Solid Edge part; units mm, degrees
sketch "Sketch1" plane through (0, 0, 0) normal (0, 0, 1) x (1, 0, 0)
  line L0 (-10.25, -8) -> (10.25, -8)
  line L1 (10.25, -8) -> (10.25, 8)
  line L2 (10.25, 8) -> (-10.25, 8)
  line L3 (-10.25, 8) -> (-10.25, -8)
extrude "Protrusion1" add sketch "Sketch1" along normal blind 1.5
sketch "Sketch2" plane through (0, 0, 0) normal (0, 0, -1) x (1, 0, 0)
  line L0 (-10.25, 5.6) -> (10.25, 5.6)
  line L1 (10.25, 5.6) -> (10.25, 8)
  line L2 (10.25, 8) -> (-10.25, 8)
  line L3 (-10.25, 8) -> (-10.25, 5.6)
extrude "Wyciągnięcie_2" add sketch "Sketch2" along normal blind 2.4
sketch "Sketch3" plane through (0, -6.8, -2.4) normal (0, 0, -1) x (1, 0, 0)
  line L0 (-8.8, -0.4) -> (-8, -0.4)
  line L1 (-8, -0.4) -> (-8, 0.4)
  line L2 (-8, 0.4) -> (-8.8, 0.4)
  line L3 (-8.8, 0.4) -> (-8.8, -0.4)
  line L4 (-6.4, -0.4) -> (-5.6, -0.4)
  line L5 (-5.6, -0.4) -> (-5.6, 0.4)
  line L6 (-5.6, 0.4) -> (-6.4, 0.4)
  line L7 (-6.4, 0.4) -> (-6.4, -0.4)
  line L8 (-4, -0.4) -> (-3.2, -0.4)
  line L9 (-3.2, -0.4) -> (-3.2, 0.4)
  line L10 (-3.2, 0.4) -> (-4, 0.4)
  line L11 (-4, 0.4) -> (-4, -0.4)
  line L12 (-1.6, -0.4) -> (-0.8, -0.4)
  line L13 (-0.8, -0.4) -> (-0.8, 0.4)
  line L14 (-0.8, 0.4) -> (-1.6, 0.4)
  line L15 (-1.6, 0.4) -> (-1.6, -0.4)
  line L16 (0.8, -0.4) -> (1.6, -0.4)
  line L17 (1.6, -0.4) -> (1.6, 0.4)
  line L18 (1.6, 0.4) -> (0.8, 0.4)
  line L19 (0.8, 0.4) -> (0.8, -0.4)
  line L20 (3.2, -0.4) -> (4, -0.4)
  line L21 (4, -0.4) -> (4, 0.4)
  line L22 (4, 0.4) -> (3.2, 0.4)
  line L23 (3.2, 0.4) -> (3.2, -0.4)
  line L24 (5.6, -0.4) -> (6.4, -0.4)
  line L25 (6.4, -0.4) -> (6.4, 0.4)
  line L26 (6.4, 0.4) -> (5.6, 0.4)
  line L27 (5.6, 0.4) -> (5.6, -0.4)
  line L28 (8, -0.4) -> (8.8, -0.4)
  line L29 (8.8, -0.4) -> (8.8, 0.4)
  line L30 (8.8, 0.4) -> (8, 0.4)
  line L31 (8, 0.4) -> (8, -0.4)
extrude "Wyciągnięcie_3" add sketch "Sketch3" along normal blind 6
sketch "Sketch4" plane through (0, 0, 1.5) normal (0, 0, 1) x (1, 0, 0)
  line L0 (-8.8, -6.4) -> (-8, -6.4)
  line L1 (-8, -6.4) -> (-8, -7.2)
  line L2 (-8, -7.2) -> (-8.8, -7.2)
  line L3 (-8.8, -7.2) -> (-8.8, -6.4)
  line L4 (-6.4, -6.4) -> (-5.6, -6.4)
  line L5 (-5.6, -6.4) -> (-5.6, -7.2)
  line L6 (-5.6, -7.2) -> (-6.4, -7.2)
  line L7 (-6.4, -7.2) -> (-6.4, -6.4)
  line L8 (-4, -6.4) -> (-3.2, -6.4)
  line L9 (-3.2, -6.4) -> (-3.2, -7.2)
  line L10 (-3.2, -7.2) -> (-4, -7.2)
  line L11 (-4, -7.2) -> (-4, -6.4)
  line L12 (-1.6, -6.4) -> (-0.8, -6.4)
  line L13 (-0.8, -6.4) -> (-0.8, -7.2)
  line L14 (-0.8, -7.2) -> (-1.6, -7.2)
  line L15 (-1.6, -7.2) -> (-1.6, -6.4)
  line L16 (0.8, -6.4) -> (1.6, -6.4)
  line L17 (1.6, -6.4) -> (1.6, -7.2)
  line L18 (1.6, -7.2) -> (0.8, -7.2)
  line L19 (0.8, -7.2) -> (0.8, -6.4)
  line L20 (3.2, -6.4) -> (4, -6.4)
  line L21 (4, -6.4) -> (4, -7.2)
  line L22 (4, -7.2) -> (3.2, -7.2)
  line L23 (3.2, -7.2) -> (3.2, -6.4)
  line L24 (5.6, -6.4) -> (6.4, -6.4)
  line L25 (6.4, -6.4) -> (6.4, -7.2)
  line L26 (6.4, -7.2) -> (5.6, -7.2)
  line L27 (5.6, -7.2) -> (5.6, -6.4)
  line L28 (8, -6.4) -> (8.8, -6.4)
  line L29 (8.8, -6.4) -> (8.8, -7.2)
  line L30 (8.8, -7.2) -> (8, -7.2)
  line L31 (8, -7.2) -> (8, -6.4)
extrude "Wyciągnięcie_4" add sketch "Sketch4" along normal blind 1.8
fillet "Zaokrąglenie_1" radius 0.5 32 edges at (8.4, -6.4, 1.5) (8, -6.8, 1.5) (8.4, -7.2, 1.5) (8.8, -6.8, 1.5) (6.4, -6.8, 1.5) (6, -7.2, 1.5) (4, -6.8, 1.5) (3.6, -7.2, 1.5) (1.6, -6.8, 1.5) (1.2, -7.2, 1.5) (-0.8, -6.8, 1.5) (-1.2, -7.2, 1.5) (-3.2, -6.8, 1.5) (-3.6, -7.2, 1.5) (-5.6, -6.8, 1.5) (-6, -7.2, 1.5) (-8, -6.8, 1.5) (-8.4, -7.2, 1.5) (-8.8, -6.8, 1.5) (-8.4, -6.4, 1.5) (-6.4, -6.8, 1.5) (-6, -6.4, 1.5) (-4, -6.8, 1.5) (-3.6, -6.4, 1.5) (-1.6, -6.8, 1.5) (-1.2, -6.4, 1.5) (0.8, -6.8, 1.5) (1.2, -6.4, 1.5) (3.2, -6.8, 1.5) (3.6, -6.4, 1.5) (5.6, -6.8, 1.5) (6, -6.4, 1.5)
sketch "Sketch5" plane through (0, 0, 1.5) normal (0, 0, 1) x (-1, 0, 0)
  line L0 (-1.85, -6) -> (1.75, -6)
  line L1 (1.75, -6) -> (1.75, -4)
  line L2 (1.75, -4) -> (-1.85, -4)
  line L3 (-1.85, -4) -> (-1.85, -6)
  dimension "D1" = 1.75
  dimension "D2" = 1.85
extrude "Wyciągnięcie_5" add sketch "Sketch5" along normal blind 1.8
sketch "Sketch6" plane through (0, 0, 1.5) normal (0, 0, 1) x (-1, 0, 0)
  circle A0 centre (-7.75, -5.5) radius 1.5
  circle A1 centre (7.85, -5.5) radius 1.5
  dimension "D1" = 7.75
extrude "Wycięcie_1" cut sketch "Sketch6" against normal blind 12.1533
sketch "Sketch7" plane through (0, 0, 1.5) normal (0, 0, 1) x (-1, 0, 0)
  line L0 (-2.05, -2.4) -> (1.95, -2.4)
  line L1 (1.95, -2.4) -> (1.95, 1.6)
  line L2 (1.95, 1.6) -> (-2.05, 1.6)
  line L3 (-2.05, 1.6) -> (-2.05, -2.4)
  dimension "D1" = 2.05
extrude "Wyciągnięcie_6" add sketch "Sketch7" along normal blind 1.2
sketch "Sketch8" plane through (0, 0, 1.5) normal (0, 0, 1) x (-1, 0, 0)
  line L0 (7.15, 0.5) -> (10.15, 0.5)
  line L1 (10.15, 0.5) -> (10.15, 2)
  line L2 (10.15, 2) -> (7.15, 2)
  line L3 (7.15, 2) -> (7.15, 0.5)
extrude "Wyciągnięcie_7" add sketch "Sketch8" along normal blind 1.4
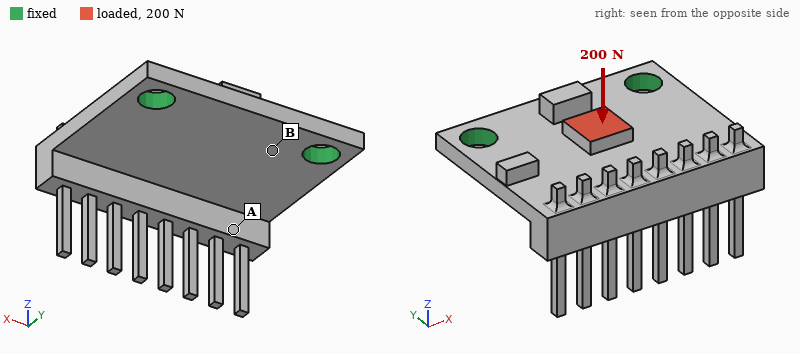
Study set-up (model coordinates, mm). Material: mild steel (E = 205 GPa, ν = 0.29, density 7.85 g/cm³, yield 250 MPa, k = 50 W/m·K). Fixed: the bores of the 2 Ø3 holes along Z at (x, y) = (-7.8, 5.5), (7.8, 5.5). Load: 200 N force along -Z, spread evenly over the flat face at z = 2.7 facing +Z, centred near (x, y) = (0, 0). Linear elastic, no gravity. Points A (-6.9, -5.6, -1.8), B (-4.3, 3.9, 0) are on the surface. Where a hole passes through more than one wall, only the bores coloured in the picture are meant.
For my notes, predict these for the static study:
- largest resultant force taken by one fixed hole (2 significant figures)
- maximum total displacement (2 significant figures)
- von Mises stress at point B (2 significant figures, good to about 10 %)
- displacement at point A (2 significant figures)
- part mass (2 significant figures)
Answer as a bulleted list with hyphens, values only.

- 100 N
- 33 µm
- 61 MPa
- 22 µm
- 5.3 g
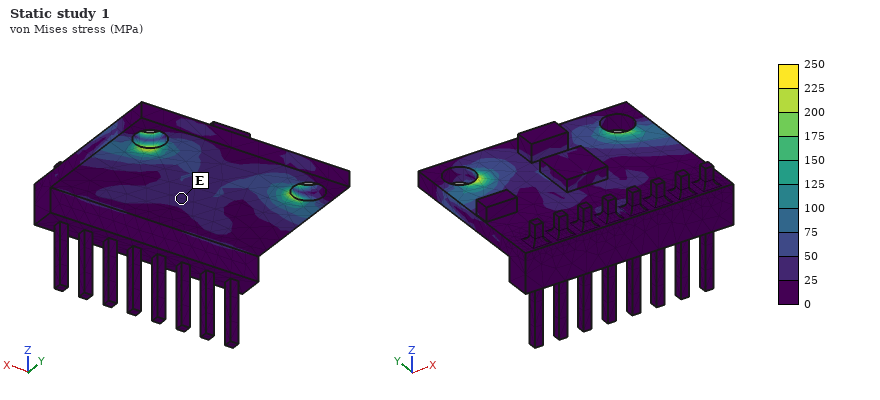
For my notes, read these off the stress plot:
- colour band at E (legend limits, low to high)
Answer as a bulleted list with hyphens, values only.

- 25 to 50 MPa
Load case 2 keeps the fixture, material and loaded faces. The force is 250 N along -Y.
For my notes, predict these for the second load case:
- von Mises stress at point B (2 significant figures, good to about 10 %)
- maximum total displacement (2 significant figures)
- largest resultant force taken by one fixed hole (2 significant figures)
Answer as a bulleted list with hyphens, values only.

- 39 MPa
- 24 µm
- 140 N
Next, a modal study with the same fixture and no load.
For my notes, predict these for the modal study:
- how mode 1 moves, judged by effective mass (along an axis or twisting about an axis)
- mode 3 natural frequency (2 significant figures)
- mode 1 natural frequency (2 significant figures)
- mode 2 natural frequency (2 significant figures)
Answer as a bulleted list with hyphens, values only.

- along Z
- 15 kHz
- 4700 Hz
- 10 kHz
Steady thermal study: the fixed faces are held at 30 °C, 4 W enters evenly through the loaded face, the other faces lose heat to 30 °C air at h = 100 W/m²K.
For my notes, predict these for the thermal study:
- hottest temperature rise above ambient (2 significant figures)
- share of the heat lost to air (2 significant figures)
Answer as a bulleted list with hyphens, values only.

- 27 K
- 25 %
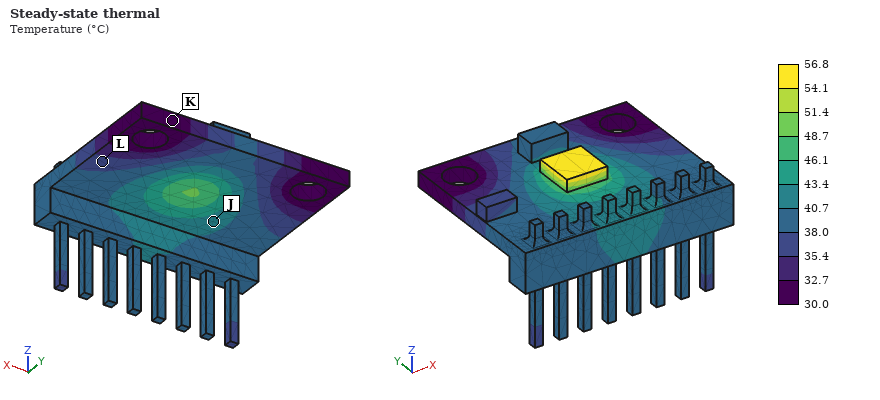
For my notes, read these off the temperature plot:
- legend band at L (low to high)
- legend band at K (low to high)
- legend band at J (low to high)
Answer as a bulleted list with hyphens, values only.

- 35.4 to 38.0 °C
- 30.0 to 32.7 °C
- 40.7 to 43.4 °C
